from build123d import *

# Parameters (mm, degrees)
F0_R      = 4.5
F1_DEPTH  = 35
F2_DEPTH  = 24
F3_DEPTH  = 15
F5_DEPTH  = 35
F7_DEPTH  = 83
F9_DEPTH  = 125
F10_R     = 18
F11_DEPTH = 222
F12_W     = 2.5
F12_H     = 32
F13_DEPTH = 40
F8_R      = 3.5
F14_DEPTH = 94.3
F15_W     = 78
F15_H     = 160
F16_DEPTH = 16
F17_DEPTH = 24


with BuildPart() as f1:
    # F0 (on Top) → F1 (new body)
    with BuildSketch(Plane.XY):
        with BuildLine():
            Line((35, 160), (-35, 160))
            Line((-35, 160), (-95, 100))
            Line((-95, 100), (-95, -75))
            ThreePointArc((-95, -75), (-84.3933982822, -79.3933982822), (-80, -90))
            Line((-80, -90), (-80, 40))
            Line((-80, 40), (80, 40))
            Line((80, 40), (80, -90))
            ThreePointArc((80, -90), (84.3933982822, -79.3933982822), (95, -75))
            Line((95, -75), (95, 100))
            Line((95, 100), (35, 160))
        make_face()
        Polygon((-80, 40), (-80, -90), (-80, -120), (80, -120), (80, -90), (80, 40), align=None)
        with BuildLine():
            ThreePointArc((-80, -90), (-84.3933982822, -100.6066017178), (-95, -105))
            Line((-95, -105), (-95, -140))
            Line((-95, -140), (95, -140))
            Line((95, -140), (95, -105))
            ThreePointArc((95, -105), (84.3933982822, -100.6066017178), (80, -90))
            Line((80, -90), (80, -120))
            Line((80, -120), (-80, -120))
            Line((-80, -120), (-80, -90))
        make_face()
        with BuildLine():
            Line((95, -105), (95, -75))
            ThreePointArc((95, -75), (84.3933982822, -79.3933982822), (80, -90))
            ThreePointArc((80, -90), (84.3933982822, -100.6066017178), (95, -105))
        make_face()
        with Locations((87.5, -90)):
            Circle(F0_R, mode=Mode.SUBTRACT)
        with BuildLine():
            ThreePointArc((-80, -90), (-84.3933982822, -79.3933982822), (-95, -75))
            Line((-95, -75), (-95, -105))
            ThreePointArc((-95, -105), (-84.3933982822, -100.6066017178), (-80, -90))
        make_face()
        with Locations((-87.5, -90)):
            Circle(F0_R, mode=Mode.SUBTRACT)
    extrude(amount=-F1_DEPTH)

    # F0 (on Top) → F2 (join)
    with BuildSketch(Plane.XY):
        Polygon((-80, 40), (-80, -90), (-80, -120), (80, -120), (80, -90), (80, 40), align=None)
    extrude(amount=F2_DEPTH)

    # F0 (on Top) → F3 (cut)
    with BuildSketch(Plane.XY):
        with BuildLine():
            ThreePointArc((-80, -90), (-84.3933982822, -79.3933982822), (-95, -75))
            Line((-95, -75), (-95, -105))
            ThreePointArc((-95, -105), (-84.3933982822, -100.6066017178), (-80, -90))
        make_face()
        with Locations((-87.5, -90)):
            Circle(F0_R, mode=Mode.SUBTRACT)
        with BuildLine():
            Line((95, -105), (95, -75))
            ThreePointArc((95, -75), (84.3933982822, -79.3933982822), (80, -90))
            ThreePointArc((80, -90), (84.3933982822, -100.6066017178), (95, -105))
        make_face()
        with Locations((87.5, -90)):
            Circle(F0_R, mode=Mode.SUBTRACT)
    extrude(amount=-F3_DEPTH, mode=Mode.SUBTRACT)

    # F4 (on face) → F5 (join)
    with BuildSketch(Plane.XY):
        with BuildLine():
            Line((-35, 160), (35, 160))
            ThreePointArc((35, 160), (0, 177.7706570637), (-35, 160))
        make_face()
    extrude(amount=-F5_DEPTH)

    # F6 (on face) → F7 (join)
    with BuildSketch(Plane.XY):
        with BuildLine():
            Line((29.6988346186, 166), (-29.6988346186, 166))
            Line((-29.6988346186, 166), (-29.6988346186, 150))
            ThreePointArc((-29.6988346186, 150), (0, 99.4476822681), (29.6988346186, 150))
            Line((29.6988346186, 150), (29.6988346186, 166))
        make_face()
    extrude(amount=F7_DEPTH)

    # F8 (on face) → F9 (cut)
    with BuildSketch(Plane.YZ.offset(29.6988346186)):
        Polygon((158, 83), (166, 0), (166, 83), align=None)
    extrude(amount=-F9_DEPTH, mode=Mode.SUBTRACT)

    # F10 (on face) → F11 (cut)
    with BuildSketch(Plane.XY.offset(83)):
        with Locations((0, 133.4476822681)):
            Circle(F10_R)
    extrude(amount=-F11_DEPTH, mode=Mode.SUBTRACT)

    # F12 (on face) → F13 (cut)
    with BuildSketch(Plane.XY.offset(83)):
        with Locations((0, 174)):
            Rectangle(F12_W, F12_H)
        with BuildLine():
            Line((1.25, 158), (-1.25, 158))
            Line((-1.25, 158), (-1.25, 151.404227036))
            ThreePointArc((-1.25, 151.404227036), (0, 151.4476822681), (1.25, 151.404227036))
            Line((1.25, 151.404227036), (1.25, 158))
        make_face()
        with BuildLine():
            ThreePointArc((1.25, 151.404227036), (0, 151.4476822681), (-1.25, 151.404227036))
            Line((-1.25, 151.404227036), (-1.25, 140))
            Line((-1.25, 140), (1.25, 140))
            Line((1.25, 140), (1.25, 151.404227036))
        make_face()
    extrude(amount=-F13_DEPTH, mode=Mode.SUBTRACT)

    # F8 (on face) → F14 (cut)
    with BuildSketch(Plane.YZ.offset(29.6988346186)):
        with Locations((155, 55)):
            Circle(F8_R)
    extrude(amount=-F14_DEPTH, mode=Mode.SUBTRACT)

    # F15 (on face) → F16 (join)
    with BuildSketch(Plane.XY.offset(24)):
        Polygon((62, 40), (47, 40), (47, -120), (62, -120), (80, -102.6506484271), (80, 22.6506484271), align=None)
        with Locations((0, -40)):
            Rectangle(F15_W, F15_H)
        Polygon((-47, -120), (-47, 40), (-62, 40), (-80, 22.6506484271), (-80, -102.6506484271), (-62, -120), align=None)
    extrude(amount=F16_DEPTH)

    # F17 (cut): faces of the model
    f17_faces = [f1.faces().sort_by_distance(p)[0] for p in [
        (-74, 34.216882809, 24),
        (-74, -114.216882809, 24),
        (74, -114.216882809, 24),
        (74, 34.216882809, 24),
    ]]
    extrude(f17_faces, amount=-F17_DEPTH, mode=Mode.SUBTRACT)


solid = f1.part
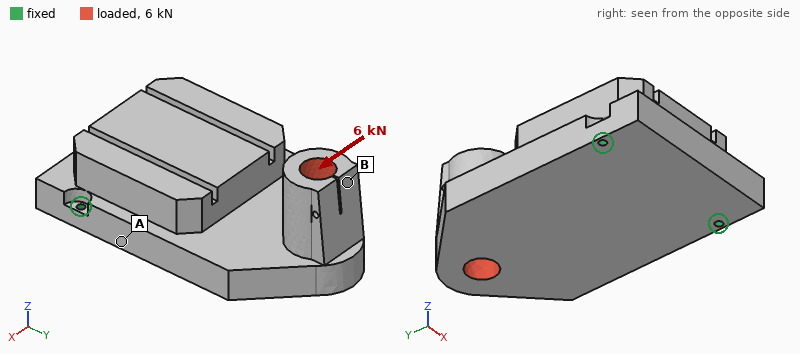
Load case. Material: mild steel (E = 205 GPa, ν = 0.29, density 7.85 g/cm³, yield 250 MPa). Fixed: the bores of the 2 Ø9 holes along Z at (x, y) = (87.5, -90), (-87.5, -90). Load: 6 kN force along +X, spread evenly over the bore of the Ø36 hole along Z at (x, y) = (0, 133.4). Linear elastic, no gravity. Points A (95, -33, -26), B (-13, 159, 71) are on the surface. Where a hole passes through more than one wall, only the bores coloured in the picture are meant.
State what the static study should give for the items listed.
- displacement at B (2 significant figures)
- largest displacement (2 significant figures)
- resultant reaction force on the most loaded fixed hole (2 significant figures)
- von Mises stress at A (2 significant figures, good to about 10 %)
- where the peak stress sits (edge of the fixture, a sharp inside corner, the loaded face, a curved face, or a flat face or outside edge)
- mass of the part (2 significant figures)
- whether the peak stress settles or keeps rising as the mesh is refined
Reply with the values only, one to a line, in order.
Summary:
26 µm
29 µm
8.4 kN
4.7 MPa
edge of the fixture
24 kg
keeps rising
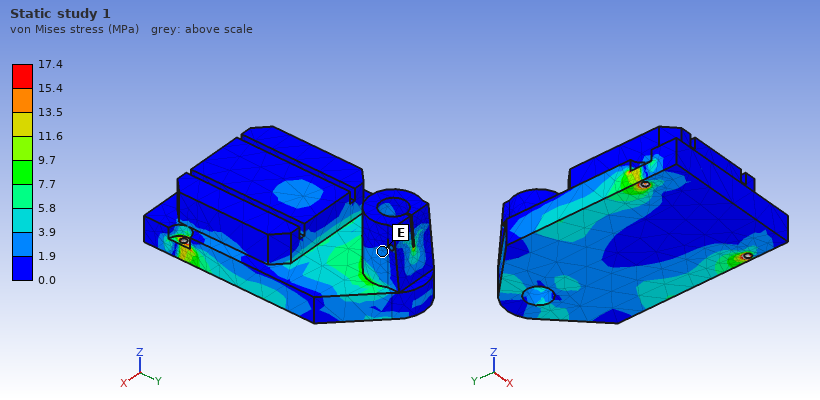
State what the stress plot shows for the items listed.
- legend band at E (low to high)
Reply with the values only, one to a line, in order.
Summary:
1.9 to 3.9 MPa
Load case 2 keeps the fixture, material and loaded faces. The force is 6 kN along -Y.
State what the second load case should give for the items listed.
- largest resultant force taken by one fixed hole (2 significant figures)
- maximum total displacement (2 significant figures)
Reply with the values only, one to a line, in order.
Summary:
3.0 kN
0.11 mm
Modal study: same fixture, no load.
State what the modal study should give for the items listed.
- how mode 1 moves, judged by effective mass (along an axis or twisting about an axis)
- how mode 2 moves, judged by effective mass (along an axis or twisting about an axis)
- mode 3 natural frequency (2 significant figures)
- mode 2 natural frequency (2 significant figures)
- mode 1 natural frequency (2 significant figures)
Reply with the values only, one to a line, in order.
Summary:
along Z
along X
1600 Hz
1400 Hz
250 Hz
